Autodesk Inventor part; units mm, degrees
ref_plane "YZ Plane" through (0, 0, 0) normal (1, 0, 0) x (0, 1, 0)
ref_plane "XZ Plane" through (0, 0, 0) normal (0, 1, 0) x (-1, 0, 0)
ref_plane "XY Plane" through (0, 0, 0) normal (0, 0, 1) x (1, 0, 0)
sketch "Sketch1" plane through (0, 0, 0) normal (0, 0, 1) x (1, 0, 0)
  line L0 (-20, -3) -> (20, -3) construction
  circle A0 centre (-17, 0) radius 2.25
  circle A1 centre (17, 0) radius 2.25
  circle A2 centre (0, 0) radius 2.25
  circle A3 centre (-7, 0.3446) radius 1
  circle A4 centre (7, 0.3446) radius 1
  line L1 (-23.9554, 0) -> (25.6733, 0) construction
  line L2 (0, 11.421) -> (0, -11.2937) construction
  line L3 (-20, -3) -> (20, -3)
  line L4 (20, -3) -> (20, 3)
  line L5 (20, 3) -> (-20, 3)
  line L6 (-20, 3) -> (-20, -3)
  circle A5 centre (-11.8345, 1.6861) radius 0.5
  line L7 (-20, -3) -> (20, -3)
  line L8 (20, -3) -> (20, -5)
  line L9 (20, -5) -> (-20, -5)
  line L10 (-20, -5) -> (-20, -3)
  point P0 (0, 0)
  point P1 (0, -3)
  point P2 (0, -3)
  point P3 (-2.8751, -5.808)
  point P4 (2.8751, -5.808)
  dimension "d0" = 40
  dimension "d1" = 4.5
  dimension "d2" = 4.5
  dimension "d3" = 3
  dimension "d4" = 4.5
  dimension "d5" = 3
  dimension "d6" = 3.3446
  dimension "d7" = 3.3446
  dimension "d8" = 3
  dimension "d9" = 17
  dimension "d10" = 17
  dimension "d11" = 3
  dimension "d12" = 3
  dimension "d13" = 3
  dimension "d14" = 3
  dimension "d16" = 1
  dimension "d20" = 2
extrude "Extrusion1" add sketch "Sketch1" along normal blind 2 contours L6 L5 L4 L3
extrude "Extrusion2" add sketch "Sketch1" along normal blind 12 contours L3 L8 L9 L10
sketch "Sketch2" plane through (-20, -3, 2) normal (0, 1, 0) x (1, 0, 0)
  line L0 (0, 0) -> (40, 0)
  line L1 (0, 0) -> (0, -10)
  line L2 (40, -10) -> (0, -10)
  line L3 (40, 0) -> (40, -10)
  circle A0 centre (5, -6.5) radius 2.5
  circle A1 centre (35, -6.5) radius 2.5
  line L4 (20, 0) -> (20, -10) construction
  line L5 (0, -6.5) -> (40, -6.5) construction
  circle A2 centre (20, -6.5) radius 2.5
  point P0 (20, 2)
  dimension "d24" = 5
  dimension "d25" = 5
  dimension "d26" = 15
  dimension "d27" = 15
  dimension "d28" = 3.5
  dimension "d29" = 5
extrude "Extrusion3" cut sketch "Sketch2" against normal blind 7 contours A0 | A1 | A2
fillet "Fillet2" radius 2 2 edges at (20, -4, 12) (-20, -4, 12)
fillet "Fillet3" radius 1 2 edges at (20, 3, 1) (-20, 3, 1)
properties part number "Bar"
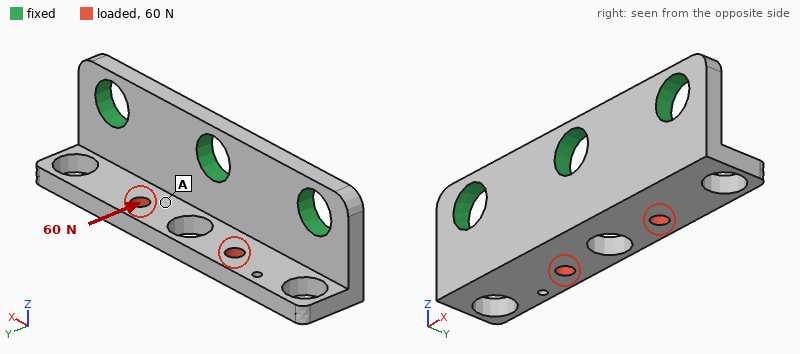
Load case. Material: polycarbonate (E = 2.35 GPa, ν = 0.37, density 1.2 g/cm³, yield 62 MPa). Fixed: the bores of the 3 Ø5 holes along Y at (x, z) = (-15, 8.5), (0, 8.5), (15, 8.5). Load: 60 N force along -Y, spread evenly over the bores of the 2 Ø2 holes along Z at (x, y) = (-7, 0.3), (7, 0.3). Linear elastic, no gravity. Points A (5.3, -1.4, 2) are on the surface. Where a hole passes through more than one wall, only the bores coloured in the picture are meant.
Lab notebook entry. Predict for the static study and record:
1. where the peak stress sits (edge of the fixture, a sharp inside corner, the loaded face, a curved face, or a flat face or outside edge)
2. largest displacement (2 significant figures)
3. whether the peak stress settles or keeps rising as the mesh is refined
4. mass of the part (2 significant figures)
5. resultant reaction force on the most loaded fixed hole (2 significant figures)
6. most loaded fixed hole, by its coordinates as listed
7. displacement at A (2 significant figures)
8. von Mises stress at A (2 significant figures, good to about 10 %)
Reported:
edge of the fixture
0.16 mm
keeps rising
1.5 g
30 N
(0, 8.5)
0.083 mm
2.8 MPa
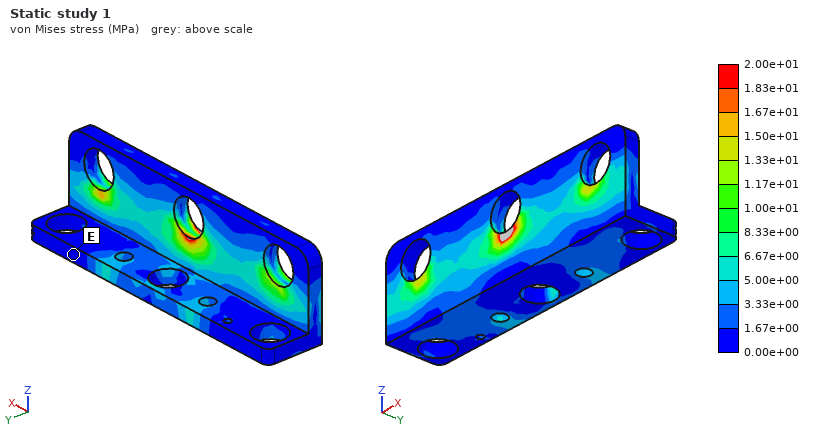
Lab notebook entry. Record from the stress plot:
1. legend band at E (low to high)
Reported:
0.00e+00 to 1.67e+00 MPa
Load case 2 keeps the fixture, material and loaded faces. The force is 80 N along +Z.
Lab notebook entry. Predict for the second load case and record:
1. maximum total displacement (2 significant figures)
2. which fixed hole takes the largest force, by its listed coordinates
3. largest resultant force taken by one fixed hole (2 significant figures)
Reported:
0.35 mm
(0, 8.5)
49 N
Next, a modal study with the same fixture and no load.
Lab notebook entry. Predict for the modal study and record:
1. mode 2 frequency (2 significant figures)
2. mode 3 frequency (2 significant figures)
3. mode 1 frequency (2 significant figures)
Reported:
4900 Hz
8200 Hz
4100 Hz
